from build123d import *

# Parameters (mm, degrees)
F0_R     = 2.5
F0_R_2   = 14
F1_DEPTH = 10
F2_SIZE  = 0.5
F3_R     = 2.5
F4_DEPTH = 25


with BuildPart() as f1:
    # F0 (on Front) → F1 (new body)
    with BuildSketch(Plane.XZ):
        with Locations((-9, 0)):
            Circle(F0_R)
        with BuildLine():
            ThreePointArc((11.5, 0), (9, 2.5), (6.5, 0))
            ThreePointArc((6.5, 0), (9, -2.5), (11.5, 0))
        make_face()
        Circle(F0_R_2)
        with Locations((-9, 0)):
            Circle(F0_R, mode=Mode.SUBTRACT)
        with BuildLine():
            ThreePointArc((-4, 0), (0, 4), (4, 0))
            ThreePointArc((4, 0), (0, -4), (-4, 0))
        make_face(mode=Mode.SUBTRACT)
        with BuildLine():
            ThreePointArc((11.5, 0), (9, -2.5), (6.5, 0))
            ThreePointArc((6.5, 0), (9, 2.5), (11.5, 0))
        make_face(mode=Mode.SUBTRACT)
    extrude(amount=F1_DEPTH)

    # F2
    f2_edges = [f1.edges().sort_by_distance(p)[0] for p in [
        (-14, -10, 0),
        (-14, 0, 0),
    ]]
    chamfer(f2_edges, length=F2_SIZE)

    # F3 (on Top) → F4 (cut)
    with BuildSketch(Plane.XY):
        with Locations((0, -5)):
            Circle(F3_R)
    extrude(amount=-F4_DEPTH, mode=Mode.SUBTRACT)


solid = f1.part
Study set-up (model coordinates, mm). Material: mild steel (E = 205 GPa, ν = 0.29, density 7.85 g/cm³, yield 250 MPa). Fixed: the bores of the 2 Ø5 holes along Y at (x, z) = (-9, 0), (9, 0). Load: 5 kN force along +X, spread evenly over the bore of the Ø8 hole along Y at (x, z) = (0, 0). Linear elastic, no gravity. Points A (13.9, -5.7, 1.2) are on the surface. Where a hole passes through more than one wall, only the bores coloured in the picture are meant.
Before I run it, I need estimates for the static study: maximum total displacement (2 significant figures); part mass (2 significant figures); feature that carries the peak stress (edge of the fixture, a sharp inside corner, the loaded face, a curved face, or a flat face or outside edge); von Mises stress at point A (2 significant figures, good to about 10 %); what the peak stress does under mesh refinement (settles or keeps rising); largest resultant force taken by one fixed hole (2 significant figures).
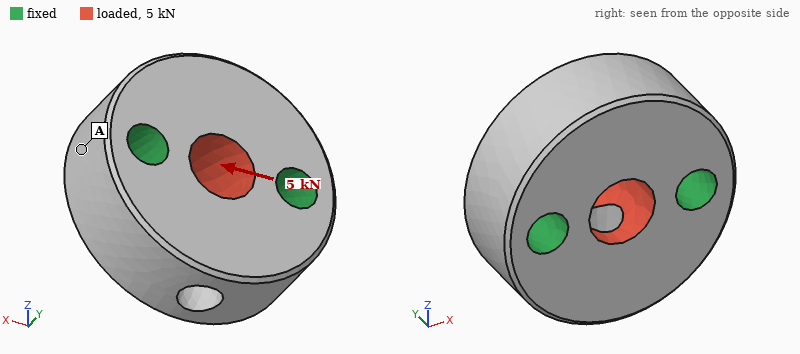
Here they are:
1.0 µm
40 g
edge of the fixture
7.5 MPa
keeps rising
2.5 kN
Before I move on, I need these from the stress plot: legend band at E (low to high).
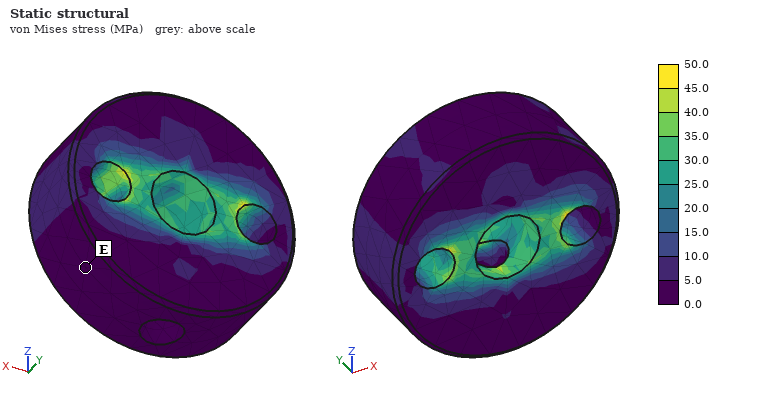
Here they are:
0.0 to 5.0 MPa
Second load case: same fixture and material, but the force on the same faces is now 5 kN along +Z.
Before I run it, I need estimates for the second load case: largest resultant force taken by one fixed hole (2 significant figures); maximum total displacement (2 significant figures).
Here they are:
2.5 kN
1.3 µm
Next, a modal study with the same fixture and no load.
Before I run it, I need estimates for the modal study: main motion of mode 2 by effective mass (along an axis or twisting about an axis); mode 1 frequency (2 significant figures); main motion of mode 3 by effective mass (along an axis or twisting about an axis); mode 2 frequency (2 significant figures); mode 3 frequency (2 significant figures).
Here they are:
along Y
39 kHz
twisting about Y
42 kHz
59 kHz
